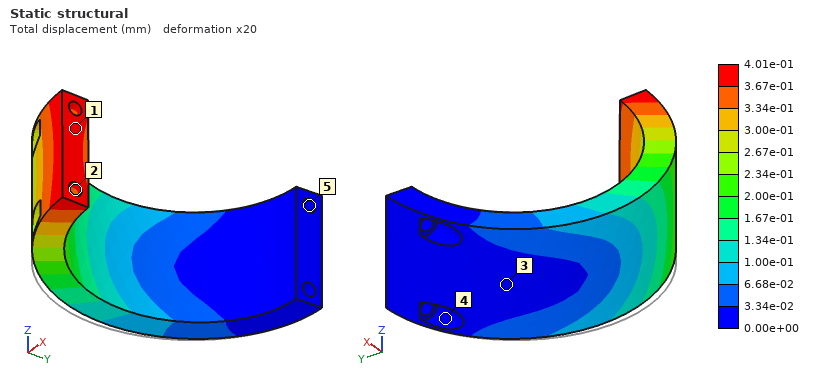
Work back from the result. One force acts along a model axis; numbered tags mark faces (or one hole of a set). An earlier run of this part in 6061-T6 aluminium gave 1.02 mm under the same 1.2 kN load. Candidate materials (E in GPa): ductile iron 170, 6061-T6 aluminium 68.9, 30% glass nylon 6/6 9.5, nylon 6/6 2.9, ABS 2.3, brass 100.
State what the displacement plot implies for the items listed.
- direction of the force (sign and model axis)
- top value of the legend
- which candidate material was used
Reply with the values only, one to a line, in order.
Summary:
+Z
4.01e-01 mm
ductile iron
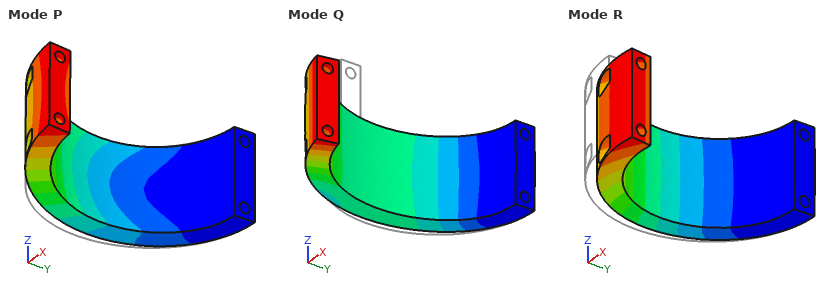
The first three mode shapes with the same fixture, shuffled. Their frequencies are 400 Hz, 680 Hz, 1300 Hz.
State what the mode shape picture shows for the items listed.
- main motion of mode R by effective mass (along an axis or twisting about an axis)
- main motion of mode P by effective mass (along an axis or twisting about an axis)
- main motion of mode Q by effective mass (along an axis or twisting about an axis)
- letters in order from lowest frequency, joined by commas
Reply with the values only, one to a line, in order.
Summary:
along X
along Z
along Y
R, P, Q
